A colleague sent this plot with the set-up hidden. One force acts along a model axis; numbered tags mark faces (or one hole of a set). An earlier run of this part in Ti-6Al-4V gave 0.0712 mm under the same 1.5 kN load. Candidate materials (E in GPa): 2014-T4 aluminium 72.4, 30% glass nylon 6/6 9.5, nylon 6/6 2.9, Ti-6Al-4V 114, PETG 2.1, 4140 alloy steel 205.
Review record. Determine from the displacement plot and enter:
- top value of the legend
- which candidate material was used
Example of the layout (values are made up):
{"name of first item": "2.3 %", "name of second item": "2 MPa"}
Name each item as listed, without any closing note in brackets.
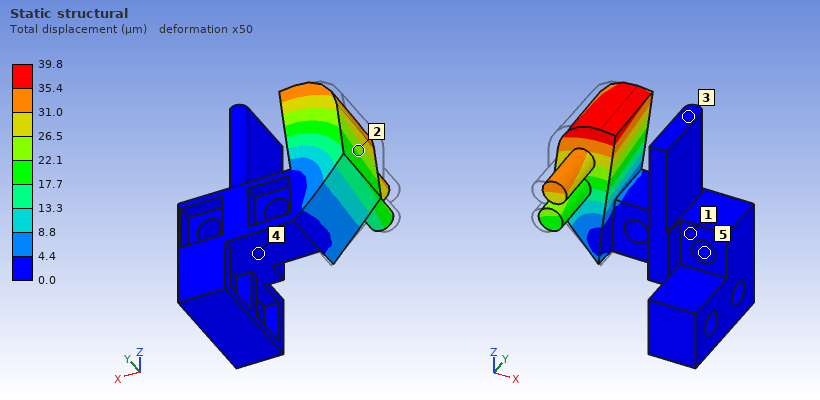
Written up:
{"top value of the legend": "39.8 µm", "which candidate material was used": "4140 alloy steel"}
